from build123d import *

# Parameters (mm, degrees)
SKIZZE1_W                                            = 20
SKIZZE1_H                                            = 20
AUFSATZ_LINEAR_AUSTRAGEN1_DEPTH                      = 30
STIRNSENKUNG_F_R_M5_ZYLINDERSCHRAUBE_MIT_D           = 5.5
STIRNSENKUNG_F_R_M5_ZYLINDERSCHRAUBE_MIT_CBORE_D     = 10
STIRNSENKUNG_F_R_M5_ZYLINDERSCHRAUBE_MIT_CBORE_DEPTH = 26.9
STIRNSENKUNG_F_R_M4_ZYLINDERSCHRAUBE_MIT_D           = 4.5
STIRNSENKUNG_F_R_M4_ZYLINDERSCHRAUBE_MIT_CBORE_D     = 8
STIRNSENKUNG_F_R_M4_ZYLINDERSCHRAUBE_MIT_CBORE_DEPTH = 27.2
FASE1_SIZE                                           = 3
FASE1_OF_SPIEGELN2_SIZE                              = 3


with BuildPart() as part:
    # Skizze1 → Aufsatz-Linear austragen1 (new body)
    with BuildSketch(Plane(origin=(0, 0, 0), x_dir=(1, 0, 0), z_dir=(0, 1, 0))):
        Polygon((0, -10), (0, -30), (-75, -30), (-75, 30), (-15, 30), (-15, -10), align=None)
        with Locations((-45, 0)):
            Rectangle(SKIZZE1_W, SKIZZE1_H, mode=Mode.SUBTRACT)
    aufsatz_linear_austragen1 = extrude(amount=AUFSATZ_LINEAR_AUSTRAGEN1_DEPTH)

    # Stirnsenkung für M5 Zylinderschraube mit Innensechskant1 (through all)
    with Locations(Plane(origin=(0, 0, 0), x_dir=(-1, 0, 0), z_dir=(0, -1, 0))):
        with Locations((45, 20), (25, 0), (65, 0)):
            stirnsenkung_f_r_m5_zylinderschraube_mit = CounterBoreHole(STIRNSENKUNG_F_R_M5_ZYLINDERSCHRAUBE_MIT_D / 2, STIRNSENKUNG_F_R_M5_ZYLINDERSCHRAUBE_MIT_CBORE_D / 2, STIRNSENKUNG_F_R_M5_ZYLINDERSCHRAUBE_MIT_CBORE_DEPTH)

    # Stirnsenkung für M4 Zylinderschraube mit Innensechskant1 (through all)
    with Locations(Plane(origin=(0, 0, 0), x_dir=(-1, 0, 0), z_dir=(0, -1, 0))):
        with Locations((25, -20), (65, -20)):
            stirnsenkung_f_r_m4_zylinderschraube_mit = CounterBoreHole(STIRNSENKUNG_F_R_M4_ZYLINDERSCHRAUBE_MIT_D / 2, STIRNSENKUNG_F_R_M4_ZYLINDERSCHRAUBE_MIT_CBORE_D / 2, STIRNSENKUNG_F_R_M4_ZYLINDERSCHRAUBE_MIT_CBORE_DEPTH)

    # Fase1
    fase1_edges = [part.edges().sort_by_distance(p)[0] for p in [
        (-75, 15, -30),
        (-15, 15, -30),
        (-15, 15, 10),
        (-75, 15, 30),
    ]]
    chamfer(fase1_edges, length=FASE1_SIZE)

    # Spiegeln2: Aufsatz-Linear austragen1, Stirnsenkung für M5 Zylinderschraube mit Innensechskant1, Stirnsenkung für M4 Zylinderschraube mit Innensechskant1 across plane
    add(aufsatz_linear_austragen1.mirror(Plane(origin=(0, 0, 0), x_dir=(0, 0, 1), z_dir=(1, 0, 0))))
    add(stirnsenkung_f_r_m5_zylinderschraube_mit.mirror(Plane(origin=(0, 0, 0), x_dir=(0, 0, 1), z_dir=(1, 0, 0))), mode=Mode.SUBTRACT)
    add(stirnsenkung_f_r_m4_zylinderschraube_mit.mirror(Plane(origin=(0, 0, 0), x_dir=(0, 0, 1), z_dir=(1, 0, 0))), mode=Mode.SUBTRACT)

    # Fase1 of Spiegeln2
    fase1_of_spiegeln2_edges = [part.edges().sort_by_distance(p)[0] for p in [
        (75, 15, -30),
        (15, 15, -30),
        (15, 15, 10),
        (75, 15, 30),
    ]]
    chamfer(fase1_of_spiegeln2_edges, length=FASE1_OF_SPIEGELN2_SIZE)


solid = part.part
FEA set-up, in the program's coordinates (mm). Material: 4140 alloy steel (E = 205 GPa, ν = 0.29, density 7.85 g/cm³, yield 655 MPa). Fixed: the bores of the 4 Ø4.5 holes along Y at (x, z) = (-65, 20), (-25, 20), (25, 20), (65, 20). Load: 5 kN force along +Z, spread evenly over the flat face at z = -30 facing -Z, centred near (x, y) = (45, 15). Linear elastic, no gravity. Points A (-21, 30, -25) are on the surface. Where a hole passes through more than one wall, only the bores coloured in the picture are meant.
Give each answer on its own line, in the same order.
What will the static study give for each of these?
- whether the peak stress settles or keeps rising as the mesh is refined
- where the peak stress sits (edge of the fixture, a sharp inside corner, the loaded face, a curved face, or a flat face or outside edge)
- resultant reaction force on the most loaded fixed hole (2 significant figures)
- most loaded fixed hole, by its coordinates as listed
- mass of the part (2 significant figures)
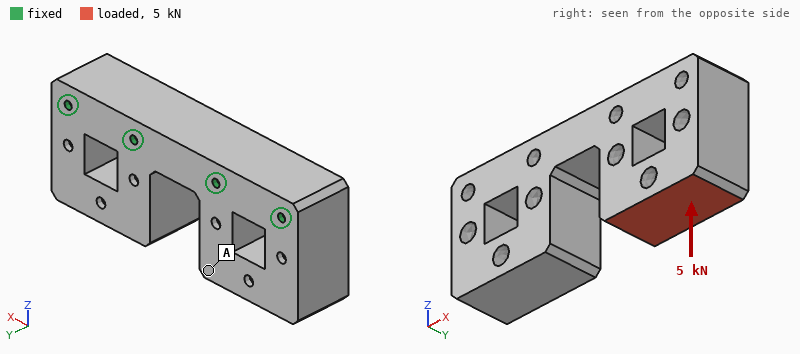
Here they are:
keeps rising
edge of the fixture
2.8 kN
(65, 20)
1.5 kg
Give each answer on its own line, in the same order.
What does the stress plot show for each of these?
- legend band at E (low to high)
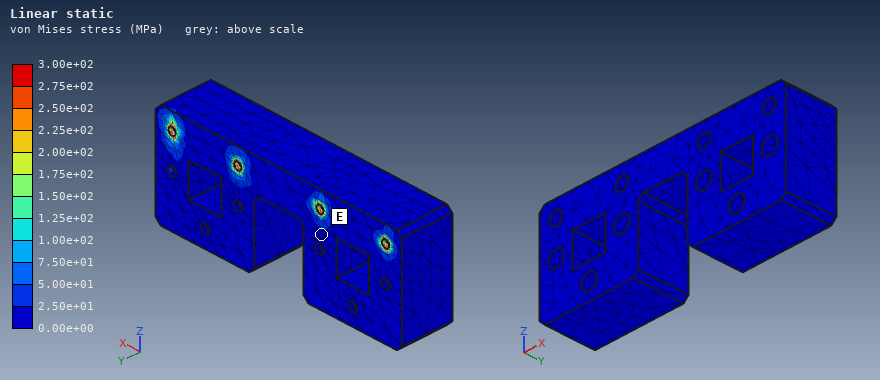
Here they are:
0.00e+00 to 2.50e+01 MPa
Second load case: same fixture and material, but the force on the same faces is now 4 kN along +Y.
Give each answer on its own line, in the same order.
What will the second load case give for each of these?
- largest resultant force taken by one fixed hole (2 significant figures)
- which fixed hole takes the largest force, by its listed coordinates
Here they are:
2.5 kN
(25, 20)
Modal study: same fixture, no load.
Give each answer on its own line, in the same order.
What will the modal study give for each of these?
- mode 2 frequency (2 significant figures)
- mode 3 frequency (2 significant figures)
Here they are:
2400 Hz
4700 Hz
